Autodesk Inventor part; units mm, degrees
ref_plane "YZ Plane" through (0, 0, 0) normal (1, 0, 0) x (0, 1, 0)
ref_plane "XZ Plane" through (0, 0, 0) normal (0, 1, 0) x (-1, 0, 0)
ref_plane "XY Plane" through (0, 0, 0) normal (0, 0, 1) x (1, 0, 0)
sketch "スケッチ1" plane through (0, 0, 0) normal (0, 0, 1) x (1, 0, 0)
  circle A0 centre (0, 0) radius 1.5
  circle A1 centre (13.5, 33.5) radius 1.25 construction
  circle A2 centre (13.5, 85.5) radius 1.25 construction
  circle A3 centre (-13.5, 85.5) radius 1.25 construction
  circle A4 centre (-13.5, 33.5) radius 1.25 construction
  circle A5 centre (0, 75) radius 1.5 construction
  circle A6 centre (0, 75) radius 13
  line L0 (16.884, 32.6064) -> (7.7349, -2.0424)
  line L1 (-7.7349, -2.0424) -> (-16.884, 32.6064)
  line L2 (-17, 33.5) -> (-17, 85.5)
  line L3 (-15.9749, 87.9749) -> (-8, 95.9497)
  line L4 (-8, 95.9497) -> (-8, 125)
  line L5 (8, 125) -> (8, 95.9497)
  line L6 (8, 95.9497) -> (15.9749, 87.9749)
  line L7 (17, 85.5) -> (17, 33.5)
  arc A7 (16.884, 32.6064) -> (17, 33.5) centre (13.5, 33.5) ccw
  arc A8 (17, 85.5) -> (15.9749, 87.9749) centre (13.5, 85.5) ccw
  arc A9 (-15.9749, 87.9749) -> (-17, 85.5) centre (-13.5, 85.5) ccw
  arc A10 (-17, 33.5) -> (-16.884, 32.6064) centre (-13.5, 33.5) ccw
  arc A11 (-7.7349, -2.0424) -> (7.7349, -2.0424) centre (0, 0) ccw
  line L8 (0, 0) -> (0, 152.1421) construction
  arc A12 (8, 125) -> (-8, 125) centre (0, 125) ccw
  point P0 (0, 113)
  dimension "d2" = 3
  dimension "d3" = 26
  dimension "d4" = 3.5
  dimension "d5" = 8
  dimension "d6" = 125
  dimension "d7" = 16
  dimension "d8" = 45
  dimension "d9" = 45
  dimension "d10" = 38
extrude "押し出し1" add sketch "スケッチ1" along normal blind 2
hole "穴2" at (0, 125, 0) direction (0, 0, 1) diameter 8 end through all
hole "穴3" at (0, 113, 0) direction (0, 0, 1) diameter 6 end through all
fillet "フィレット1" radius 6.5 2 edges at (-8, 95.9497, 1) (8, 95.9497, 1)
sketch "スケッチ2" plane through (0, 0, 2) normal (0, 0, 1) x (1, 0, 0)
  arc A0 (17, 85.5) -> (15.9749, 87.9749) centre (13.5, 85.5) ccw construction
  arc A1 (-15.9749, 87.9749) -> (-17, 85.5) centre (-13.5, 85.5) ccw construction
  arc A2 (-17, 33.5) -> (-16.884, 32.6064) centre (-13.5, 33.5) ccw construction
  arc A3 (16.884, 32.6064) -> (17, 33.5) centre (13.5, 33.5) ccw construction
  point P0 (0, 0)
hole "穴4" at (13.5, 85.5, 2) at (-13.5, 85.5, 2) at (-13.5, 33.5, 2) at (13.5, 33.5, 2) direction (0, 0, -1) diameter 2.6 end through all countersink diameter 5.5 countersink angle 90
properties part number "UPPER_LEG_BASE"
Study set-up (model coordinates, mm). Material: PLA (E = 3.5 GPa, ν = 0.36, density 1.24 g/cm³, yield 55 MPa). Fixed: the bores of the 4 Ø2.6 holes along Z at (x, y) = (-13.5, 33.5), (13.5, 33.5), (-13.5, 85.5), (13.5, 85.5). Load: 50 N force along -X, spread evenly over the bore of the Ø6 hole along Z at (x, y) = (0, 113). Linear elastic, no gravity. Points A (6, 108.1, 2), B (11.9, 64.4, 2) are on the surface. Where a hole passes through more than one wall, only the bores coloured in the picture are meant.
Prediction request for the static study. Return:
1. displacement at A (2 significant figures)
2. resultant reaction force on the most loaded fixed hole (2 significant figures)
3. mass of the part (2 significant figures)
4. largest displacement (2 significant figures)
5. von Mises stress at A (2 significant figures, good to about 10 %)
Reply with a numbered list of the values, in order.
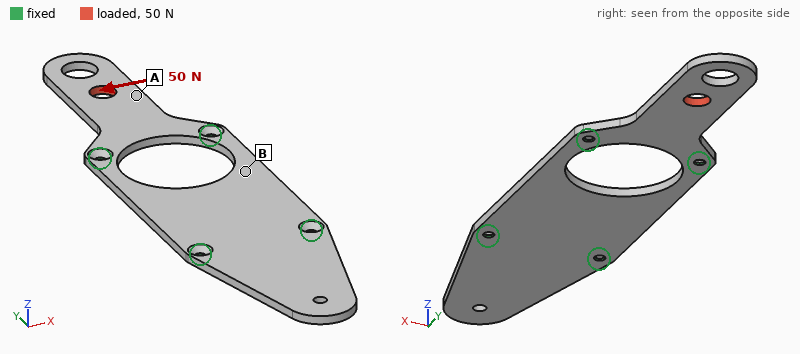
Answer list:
1. 0.10 mm
2. 57 N
3. 7.2 g
4. 0.27 mm
5. 2.8 MPa
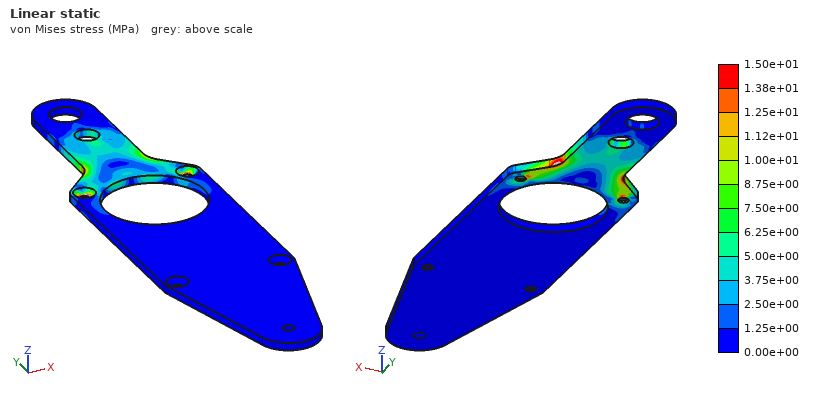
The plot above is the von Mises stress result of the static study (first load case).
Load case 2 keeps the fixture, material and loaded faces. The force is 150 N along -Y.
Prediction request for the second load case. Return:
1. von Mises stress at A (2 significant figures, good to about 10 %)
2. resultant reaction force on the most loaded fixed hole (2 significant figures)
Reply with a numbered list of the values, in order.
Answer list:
1. 4.7 MPa
2. 85 N
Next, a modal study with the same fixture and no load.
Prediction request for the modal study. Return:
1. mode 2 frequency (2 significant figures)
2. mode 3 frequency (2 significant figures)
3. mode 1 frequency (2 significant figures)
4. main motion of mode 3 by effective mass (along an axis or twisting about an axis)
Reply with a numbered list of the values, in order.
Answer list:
1. 350 Hz
2. 940 Hz
3. 240 Hz
4. along Z
